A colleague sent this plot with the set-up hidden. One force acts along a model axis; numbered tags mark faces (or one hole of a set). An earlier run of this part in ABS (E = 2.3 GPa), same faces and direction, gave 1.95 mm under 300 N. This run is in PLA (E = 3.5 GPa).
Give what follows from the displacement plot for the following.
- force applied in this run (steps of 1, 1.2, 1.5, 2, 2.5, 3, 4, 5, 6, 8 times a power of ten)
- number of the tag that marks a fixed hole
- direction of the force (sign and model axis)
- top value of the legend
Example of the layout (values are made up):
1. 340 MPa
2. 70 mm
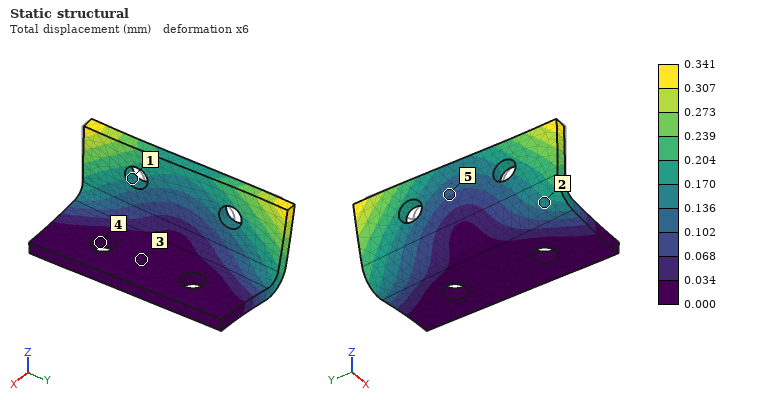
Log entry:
1. 80 N
2. 4
3. +Y
4. 0.341 mm
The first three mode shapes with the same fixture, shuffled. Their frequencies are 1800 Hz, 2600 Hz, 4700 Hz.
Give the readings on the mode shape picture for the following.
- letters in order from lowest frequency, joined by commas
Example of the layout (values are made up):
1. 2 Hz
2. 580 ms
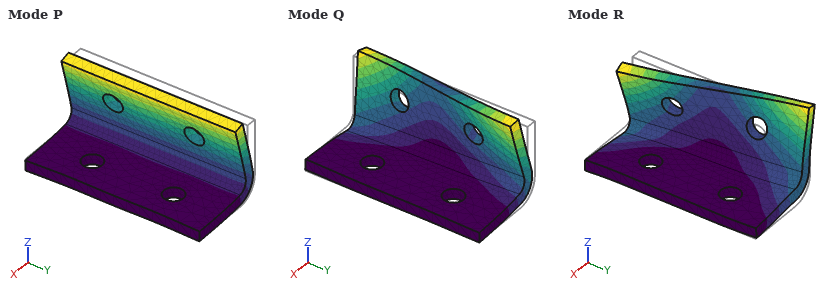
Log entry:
1. P, Q, R
